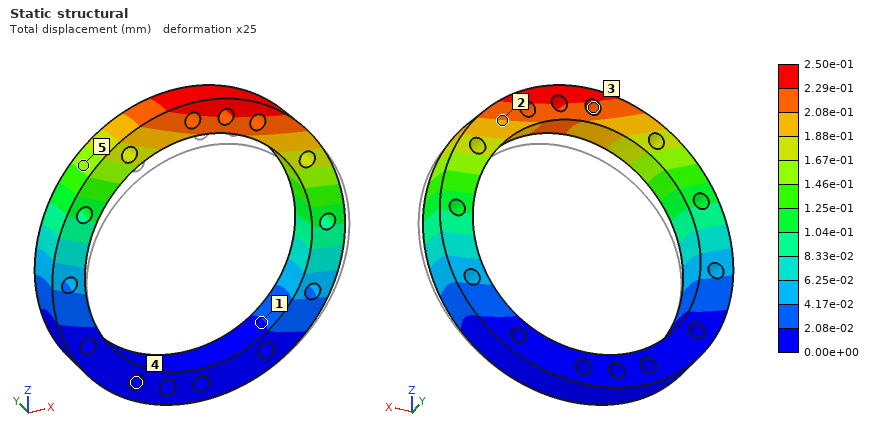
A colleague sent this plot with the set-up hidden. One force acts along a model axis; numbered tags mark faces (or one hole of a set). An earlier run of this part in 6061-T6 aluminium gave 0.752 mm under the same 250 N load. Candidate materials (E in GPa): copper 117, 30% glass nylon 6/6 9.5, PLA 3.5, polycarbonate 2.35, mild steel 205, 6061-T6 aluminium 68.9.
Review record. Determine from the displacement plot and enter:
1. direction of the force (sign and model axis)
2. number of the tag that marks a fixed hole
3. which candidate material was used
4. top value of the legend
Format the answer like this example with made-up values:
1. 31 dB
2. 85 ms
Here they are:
1. +Y
2. 4
3. mild steel
4. 2.50e-01 mm
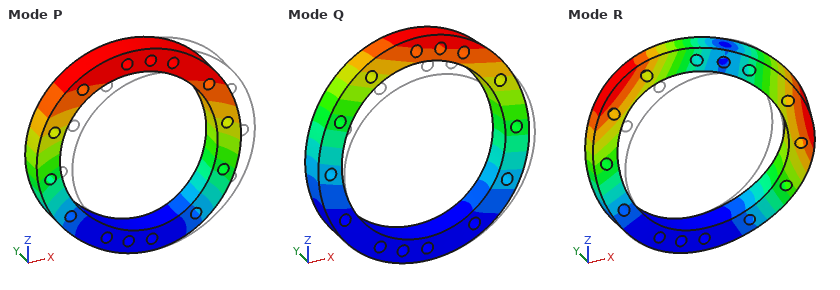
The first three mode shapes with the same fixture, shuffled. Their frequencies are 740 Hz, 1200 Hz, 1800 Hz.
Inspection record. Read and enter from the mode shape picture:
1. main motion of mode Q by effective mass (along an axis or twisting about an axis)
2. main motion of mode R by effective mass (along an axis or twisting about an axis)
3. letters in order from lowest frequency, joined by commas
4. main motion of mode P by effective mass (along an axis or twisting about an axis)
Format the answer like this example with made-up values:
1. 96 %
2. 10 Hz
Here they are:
1. along Y
2. twisting about Z
3. Q, P, R
4. along X
